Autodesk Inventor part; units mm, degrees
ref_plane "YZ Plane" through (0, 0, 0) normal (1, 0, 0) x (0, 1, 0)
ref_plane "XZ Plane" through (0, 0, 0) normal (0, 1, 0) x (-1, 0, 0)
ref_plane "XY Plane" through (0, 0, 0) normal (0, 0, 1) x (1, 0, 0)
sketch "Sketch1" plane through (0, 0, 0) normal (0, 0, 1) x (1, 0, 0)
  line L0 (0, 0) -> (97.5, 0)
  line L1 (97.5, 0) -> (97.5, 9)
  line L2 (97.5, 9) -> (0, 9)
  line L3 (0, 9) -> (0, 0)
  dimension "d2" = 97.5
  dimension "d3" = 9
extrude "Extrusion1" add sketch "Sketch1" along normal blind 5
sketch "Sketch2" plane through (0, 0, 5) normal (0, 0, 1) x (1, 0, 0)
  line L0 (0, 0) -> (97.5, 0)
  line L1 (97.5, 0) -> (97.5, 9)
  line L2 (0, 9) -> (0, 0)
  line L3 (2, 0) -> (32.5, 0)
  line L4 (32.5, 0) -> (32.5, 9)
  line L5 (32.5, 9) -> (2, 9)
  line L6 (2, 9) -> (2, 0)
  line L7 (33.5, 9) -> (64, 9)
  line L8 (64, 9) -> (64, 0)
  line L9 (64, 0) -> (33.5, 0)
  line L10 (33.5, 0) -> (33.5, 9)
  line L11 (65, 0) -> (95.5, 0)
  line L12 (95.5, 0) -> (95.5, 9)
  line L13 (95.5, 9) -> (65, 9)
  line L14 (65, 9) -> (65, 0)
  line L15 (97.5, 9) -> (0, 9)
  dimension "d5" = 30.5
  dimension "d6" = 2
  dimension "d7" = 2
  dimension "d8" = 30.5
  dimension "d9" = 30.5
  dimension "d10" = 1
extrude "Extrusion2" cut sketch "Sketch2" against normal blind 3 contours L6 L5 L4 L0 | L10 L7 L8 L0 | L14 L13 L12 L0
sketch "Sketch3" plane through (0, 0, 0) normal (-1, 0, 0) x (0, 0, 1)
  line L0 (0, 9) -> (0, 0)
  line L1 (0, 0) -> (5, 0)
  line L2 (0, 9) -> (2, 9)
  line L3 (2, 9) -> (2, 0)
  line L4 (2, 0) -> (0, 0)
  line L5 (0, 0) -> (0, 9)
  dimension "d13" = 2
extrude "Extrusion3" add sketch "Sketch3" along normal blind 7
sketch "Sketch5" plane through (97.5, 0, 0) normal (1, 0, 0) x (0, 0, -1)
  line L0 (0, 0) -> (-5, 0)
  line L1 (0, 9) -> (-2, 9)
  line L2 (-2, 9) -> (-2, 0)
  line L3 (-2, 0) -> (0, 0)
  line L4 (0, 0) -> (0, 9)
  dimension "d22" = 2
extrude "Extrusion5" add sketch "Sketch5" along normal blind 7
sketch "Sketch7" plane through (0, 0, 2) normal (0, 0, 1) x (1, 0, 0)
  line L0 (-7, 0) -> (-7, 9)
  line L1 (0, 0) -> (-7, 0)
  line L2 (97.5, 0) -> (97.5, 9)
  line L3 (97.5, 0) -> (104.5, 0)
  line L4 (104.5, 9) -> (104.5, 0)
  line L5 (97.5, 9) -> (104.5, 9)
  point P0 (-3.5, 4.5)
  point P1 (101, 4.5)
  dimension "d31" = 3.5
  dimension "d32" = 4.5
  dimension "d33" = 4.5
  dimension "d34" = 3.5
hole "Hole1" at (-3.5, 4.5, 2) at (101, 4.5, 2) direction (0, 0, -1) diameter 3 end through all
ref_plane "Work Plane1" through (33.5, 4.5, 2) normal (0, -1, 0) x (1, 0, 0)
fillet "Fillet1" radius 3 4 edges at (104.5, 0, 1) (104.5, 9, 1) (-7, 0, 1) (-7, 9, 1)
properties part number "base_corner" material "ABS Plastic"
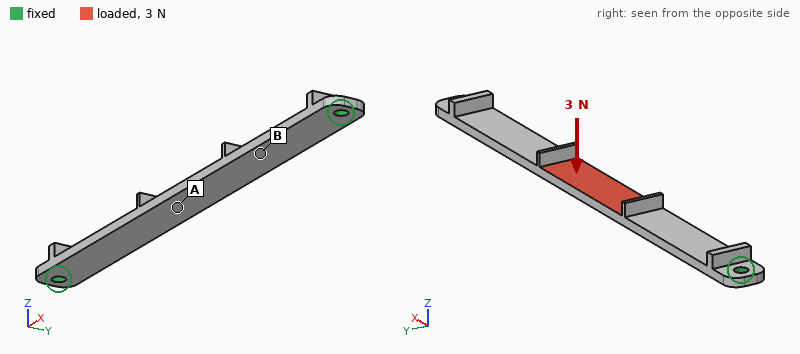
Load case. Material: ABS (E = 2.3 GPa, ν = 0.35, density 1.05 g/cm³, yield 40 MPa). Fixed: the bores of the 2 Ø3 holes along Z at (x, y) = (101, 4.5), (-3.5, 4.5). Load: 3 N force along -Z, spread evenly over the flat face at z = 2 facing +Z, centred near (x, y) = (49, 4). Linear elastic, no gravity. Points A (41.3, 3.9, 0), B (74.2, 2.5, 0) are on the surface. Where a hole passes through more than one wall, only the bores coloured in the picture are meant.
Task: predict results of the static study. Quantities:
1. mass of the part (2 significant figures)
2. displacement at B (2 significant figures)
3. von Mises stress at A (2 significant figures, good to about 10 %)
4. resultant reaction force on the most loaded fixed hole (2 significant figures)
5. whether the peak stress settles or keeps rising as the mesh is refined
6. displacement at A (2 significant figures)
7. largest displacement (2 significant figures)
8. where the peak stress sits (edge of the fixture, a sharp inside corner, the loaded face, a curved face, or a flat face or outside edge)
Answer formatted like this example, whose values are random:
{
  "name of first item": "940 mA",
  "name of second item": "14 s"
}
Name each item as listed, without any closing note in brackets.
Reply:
{
  "mass of the part": "2.2 g",
  "displacement at B": "0.57 mm",
  "von Mises stress at A": "4.1 MPa",
  "resultant reaction force on the most loaded fixed hole": "1.5 N",
  "whether the peak stress settles or keeps rising as the mesh is refined": "keeps rising",
  "displacement at A": "1.0 mm",
  "largest displacement": "1.1 mm",
  "where the peak stress sits": "edge of the fixture"
}
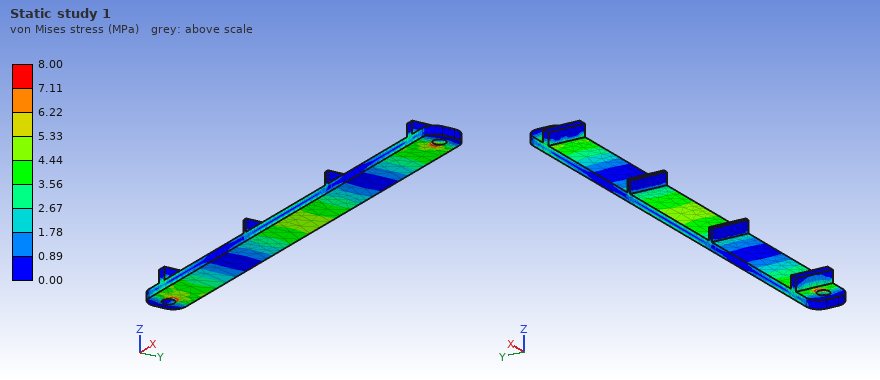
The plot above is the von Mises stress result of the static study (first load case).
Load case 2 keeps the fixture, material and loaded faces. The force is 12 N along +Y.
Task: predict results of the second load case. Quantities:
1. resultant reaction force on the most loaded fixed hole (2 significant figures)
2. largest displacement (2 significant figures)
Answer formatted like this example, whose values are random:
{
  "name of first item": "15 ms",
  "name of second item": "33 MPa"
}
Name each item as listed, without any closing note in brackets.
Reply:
{
  "resultant reaction force on the most loaded fixed hole": "6.0 N",
  "largest displacement": "0.33 mm"
}
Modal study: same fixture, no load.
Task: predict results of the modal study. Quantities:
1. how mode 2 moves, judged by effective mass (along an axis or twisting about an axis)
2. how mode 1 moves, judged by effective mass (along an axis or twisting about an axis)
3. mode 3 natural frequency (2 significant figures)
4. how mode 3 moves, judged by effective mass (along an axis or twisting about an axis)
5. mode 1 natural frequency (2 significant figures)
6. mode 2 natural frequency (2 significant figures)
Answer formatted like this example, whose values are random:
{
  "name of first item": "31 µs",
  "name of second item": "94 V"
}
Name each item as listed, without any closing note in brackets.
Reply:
{
  "how mode 2 moves, judged by effective mass": "twisting about Y",
  "how mode 1 moves, judged by effective mass": "along Z",
  "mode 3 natural frequency": "1000 Hz",
  "how mode 3 moves, judged by effective mass": "along Y",
  "mode 1 natural frequency": "290 Hz",
  "mode 2 natural frequency": "790 Hz"
}
